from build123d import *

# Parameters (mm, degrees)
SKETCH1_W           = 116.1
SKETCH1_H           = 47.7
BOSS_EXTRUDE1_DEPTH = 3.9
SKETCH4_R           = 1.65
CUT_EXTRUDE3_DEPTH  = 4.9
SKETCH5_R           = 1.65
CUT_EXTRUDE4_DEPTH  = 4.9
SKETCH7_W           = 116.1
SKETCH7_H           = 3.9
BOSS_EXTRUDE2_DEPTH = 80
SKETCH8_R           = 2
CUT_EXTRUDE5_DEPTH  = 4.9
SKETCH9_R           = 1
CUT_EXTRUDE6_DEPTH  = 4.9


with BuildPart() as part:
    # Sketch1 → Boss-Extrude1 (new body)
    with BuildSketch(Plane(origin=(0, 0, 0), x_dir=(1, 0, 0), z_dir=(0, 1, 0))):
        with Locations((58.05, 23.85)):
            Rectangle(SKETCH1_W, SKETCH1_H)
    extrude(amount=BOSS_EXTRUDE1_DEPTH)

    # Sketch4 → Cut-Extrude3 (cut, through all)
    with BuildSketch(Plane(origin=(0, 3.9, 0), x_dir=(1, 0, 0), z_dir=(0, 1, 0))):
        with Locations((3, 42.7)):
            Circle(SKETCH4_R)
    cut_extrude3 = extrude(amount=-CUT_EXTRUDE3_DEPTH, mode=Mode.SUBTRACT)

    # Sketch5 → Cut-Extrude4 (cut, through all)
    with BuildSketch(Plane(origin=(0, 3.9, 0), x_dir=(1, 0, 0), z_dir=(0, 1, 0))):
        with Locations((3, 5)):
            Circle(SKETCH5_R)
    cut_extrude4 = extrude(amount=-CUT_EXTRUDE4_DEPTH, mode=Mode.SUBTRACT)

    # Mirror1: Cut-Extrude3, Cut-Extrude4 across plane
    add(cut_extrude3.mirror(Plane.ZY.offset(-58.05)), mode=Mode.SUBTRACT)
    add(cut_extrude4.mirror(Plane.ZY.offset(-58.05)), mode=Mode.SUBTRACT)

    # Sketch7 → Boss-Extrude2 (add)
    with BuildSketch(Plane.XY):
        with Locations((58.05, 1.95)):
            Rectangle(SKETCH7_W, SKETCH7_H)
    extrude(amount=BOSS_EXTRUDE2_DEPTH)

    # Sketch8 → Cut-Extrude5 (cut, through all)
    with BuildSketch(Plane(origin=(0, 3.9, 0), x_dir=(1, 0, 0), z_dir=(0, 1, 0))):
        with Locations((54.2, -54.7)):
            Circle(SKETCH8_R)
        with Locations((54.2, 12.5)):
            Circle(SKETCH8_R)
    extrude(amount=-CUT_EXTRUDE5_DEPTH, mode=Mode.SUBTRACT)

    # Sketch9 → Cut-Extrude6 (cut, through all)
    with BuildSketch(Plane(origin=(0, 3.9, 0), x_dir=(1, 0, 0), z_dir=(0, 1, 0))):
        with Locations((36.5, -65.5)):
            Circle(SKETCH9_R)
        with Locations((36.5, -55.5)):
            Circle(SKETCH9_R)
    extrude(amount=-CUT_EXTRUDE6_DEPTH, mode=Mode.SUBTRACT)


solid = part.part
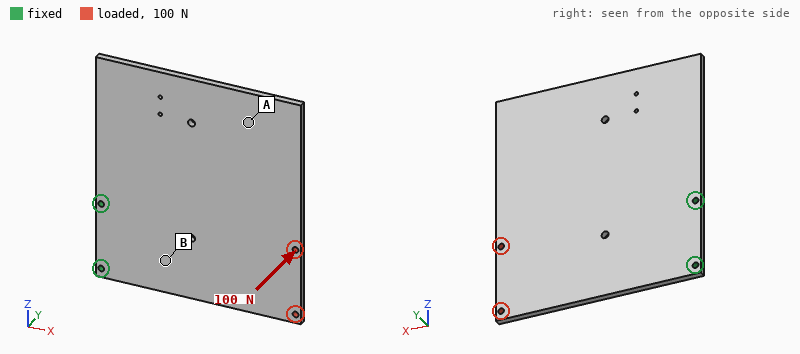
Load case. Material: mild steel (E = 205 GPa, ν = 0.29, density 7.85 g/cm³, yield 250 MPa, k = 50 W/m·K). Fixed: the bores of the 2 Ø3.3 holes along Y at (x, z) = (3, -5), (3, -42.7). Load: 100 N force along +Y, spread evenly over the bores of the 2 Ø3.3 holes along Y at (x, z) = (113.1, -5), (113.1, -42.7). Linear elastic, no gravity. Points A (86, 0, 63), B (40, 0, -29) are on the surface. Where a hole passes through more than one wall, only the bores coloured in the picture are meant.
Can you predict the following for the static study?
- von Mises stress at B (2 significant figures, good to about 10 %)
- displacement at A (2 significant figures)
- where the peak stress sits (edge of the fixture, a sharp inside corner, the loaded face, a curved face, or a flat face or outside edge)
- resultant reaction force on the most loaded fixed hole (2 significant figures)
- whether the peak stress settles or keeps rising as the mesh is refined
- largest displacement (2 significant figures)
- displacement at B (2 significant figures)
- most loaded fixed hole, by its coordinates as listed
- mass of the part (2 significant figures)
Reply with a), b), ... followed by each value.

a) 34 MPa
b) 0.39 mm
c) edge of the fixture
d) 76 N
e) keeps rising
f) 0.71 mm
g) 0.13 mm
h) (3, -5)
i) 450 g
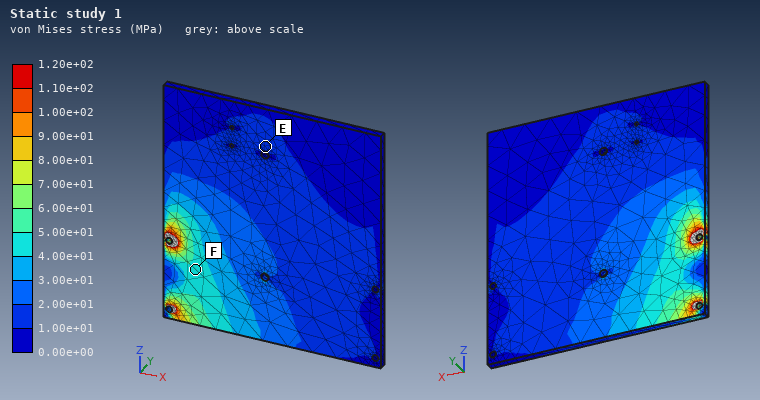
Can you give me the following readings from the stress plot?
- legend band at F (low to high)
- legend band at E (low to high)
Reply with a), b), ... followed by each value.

a) 4.00e+01 to 5.00e+01 MPa
b) 1.00e+01 to 2.00e+01 MPa
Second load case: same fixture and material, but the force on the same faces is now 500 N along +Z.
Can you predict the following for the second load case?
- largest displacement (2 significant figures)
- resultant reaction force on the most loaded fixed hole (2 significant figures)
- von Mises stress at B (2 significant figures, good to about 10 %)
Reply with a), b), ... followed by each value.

a) 31 µm
b) 1.5 kN
c) 8.8 MPa
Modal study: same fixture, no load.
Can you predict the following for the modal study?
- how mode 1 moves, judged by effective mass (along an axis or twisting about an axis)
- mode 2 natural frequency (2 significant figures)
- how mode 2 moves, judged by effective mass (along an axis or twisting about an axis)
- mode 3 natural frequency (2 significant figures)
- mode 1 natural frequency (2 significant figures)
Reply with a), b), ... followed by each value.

a) along Y
b) 330 Hz
c) twisting about X
d) 780 Hz
e) 160 Hz
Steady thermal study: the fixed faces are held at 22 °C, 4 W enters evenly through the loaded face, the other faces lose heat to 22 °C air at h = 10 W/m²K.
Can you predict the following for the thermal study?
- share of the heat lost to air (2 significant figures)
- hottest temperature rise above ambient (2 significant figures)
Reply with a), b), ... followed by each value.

a) 60 %
b) 28 K
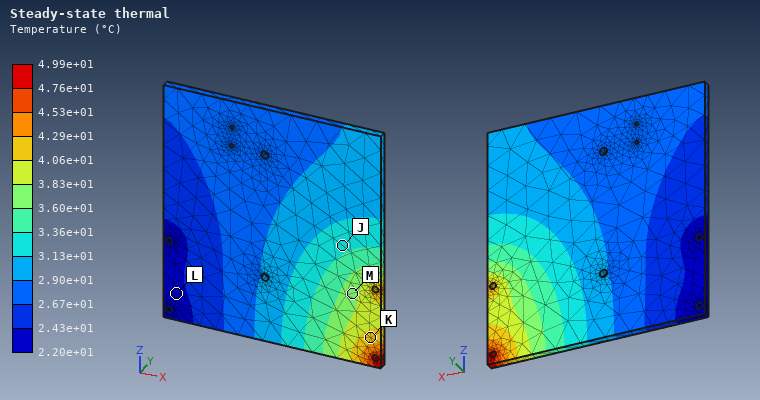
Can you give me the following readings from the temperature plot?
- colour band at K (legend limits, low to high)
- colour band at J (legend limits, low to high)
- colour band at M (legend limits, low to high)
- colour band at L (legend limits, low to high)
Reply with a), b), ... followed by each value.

a) 4.06e+01 to 4.29e+01 °C
b) 3.13e+01 to 3.36e+01 °C
c) 3.60e+01 to 3.83e+01 °C
d) 2.20e+01 to 2.43e+01 °C
